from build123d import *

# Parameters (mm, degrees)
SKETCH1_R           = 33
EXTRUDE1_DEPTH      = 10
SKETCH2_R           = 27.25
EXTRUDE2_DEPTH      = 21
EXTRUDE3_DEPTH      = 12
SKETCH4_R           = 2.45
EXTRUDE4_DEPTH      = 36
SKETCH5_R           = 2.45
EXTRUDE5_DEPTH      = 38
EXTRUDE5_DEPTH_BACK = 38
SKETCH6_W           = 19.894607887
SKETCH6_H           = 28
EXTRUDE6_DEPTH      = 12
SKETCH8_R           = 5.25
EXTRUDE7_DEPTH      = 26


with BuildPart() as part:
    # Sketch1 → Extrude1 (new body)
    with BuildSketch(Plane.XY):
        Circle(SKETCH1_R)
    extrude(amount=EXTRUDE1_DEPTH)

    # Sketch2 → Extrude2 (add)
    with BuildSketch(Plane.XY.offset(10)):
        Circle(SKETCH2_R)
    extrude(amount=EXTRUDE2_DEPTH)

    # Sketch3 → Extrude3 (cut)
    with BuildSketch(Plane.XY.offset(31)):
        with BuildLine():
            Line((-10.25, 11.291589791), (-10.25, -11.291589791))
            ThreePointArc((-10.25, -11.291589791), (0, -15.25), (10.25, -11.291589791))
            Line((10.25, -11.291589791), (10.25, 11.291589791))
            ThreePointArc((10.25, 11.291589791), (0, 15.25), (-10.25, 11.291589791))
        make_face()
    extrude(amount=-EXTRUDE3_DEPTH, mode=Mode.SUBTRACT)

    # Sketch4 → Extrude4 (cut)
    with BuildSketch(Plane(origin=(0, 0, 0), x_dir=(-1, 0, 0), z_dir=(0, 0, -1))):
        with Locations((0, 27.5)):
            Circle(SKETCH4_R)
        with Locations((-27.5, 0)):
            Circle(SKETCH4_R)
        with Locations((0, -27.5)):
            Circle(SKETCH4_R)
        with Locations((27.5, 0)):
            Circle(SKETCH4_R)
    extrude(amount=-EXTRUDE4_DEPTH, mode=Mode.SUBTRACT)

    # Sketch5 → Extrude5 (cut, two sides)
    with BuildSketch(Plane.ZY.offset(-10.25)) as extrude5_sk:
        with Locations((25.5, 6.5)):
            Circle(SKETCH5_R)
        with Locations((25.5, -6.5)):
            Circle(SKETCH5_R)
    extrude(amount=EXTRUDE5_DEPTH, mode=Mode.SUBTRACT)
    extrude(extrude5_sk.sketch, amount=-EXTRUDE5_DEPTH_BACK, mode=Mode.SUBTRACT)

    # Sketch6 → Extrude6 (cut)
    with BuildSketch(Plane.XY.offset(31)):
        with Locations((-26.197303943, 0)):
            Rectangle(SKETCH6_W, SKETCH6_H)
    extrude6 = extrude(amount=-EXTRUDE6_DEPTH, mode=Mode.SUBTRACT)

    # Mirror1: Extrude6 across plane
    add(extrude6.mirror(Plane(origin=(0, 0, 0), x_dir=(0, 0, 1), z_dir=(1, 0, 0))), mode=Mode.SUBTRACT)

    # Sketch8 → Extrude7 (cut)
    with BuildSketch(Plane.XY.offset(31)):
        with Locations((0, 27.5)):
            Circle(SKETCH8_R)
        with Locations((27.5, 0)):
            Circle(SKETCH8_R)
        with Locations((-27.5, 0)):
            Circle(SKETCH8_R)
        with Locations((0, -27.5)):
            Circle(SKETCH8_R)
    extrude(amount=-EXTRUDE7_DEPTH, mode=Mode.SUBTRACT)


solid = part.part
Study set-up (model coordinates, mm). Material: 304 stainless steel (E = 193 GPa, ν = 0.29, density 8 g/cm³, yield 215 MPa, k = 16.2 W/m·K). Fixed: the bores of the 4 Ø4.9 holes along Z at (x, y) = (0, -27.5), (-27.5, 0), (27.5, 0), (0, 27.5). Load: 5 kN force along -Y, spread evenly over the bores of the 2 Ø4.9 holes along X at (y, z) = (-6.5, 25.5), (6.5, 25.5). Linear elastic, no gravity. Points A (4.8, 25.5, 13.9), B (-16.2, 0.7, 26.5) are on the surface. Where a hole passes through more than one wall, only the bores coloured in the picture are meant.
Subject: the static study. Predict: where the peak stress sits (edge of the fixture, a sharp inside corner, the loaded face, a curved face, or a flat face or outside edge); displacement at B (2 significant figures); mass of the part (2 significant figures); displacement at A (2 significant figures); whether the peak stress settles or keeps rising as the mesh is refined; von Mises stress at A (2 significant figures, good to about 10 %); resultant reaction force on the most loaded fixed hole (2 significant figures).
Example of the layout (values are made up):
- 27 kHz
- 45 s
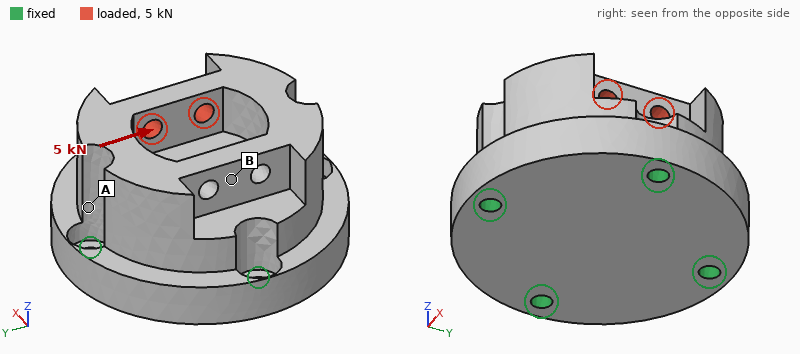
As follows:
- edge of the fixture
- 2.5 µm
- 520 g
- 3.6 µm
- keeps rising
- 15 MPa
- 2.7 kN
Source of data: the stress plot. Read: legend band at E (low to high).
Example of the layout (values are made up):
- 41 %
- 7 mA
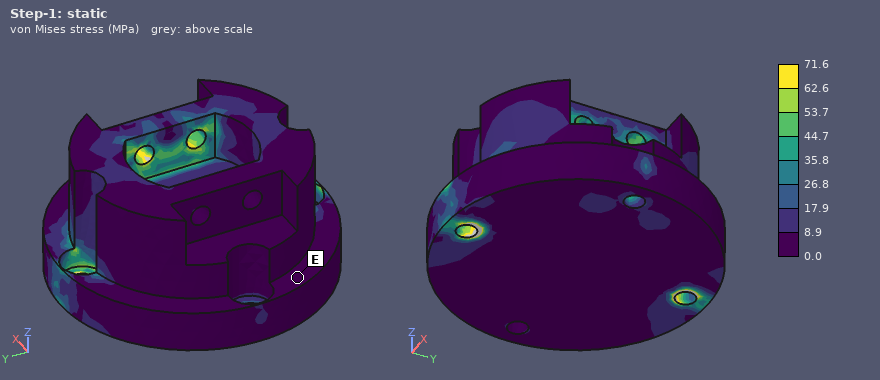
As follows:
- 0.0 to 8.9 MPa
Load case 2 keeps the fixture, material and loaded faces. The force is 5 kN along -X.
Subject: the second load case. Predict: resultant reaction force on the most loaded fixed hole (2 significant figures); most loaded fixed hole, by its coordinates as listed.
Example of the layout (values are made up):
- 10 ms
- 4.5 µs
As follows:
- 2.9 kN
- (27.5, 0)
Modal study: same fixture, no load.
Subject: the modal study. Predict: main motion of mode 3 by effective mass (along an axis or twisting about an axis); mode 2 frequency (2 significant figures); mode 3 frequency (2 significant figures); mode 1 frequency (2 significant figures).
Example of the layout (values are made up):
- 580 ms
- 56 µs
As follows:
- along Z
- 12 kHz
- 13 kHz
- 11 kHz
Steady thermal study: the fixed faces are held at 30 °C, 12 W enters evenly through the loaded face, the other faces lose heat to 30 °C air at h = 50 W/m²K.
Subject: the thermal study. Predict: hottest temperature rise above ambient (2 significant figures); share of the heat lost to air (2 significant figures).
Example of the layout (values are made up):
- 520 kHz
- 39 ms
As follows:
- 46 K
- 47 %
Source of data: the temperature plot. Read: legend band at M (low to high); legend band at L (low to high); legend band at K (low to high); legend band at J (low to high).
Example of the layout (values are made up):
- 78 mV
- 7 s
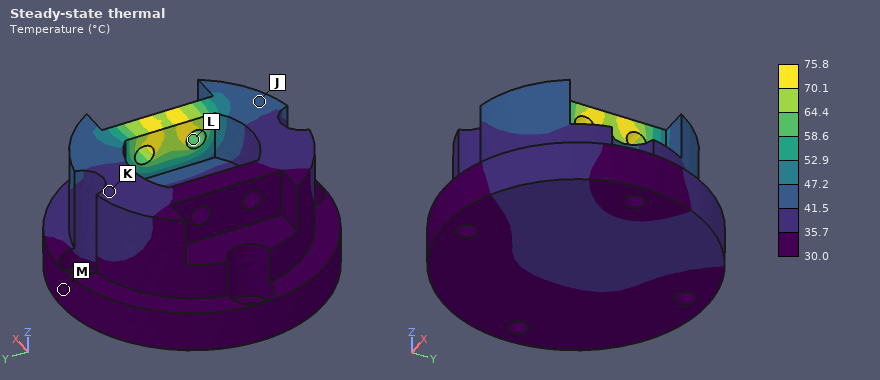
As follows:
- 30.0 to 35.7 °C
- 58.6 to 64.4 °C
- 35.7 to 41.5 °C
- 41.5 to 47.2 °C
